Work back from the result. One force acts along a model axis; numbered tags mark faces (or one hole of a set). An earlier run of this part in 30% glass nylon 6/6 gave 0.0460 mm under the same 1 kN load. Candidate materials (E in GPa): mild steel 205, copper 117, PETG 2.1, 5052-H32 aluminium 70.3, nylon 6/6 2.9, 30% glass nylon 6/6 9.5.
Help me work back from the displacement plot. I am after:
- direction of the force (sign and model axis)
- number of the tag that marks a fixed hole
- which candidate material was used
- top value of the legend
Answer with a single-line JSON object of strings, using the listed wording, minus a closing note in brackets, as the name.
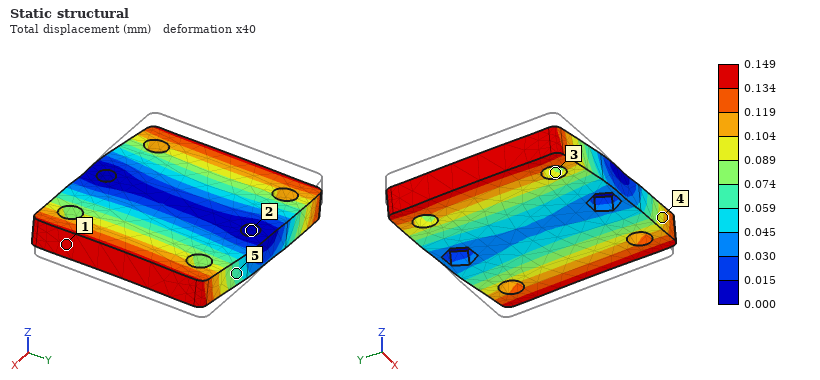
{"direction of the force": "+X", "number of the tag that marks a fixed hole": "2", "which candidate material was used": "nylon 6/6", "top value of the legend": "0.149 mm"}
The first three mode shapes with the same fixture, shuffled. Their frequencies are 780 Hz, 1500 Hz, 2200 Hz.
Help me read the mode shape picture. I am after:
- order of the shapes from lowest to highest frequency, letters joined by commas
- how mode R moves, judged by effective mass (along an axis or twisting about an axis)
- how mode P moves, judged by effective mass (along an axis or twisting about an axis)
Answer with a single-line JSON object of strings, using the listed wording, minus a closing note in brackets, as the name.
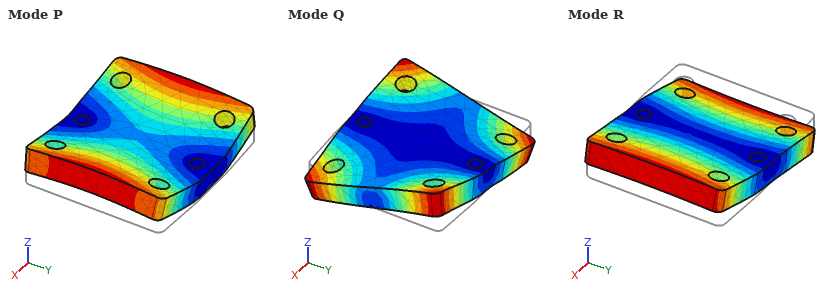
{"order of the shapes from lowest to highest frequency, letters joined by commas": "R, P, Q", "how mode R moves, judged by effective mass": "twisting about Y", "how mode P moves, judged by effective mass": "along Z"}
